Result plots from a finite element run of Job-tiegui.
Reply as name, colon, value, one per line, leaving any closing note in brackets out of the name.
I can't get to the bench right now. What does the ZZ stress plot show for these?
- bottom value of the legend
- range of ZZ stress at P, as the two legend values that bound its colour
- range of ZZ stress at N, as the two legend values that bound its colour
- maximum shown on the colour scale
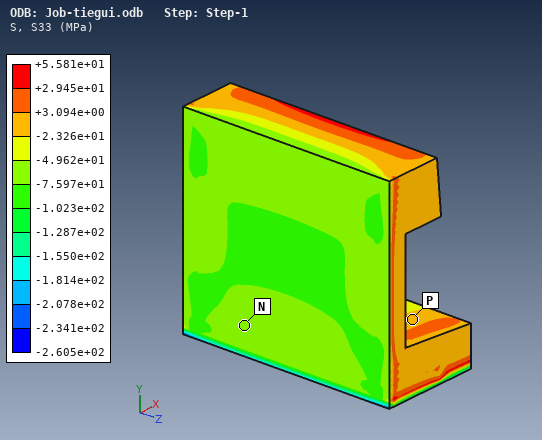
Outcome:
bottom value of the legend: -2.605e+02 MPa
range of ZZ stress at P, as the two legend values that bound its colour: -2.326e+01 to +3.094e+00 MPa
range of ZZ stress at N, as the two legend values that bound its colour: -7.597e+01 to -4.962e+01 MPa
maximum shown on the colour scale: +5.581e+01 MPa
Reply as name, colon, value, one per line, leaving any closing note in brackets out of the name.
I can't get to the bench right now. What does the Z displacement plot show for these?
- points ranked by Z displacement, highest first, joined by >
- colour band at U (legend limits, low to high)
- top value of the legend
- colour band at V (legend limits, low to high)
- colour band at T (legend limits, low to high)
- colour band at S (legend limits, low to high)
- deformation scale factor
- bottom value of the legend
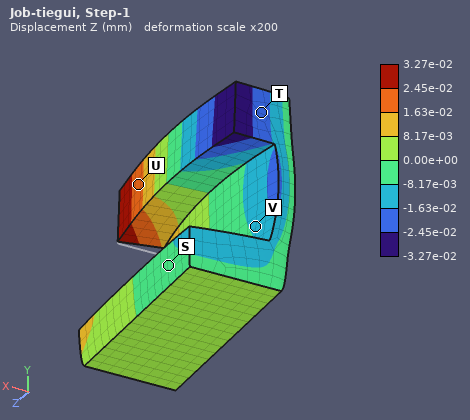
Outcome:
points ranked by Z displacement, highest first, joined by >: U > S > V > T
colour band at U: 1.63e-02 to 2.45e-02 mm
top value of the legend: 3.27e-02 mm
colour band at V: -1.63e-02 to -8.17e-03 mm
colour band at T: -2.45e-02 to -1.63e-02 mm
colour band at S: -8.17e-03 to 0.00e+00 mm
deformation scale factor: 200
bottom value of the legend: -3.27e-02 mm
